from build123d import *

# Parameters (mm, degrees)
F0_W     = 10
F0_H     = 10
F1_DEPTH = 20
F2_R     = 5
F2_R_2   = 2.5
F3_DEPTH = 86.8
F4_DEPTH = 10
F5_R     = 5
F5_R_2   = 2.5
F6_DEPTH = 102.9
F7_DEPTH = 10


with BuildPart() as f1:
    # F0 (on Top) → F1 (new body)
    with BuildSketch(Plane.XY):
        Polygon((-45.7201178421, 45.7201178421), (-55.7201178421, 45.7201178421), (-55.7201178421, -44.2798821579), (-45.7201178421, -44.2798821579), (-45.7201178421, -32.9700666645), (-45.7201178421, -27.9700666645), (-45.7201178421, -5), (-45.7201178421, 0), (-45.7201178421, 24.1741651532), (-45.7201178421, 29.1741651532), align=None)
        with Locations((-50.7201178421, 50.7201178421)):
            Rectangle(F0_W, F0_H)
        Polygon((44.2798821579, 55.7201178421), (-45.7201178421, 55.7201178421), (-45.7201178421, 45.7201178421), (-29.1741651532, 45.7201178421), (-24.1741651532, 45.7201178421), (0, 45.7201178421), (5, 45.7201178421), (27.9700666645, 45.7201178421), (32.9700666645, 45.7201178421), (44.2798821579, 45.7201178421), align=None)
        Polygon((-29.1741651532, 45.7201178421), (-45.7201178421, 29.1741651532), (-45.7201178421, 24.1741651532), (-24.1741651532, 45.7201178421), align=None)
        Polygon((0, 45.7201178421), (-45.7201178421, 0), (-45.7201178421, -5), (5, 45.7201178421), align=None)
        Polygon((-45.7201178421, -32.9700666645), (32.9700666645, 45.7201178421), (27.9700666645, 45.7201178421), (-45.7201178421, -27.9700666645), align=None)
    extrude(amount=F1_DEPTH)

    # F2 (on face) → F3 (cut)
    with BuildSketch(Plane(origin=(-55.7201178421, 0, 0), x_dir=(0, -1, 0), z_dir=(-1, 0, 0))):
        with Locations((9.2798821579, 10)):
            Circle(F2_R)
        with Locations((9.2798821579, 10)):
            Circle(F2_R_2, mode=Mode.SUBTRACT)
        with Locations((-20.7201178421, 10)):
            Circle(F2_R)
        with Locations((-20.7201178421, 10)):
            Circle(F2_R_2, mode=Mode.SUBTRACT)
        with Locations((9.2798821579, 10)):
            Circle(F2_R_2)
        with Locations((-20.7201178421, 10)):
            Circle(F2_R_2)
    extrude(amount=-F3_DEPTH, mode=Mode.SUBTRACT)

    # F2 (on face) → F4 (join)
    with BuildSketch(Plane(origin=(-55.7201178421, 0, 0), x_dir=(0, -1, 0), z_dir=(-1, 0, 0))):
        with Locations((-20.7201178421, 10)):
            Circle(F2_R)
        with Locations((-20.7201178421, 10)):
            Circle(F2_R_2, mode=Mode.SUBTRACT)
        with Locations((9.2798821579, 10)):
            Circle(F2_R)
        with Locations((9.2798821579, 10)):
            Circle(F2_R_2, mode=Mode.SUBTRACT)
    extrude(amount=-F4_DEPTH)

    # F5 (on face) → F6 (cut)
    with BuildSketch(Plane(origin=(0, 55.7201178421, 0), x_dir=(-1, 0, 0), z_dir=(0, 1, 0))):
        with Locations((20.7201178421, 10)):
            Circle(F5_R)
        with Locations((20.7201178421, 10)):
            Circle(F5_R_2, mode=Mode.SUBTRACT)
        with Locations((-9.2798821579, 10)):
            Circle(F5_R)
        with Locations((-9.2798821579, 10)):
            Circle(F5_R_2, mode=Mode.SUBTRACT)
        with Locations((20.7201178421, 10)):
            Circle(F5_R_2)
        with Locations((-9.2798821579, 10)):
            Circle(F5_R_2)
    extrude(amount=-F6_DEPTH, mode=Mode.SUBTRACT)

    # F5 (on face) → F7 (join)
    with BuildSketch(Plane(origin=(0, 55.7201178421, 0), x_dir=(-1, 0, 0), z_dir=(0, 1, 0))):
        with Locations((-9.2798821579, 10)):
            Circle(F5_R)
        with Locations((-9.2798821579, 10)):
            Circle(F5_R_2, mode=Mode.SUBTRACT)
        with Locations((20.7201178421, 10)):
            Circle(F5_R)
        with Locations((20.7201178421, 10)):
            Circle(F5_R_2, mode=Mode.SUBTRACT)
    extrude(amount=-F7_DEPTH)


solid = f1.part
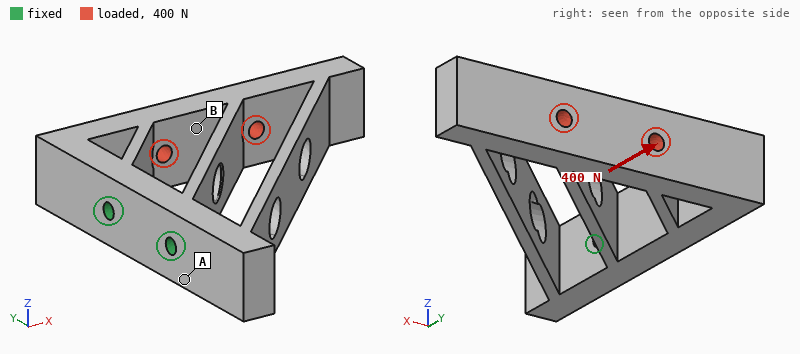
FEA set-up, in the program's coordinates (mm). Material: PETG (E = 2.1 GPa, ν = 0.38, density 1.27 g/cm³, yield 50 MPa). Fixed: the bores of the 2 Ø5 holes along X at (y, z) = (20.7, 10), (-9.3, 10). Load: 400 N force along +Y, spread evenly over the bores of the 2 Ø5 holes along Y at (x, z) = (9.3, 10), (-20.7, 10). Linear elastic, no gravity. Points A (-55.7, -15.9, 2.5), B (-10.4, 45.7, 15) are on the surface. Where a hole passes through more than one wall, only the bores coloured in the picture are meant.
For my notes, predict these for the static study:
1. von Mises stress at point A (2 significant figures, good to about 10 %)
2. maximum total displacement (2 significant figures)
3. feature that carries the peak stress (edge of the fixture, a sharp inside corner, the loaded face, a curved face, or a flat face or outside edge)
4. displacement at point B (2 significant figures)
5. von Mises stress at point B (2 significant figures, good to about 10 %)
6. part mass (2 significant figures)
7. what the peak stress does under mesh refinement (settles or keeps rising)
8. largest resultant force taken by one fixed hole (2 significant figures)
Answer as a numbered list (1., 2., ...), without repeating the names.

1. 3.0 MPa
2. 1.3 mm
3. edge of the fixture
4. 1.2 mm
5. 7.5 MPa
6. 63 g
7. keeps rising
8. 400 N
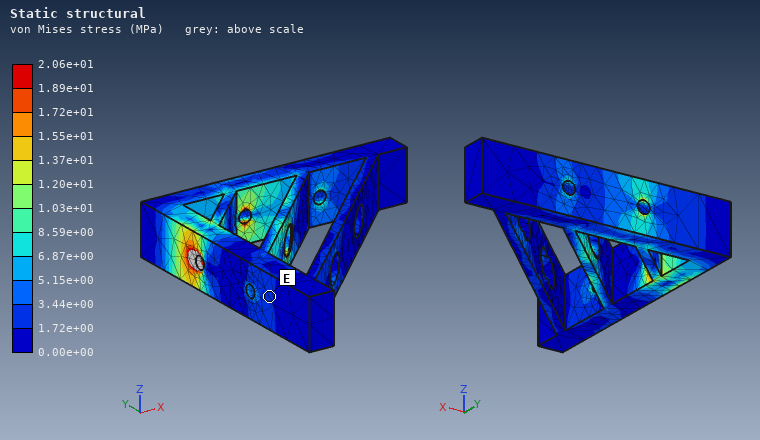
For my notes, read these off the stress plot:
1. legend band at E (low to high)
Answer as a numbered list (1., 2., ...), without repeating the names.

1. 1.72e+00 to 3.44e+00 MPa
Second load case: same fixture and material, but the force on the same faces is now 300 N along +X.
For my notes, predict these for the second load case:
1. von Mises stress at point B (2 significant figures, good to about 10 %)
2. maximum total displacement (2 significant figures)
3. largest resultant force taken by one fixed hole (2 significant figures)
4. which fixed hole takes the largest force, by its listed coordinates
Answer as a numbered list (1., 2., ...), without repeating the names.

1. 4.8 MPa
2. 0.84 mm
3. 410 N
4. (20.7, 10)
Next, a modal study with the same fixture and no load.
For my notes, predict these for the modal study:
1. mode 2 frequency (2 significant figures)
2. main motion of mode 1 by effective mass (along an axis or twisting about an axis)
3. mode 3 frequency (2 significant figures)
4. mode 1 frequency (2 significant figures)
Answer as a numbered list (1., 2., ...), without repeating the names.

1. 400 Hz
2. along Z
3. 510 Hz
4. 300 Hz
